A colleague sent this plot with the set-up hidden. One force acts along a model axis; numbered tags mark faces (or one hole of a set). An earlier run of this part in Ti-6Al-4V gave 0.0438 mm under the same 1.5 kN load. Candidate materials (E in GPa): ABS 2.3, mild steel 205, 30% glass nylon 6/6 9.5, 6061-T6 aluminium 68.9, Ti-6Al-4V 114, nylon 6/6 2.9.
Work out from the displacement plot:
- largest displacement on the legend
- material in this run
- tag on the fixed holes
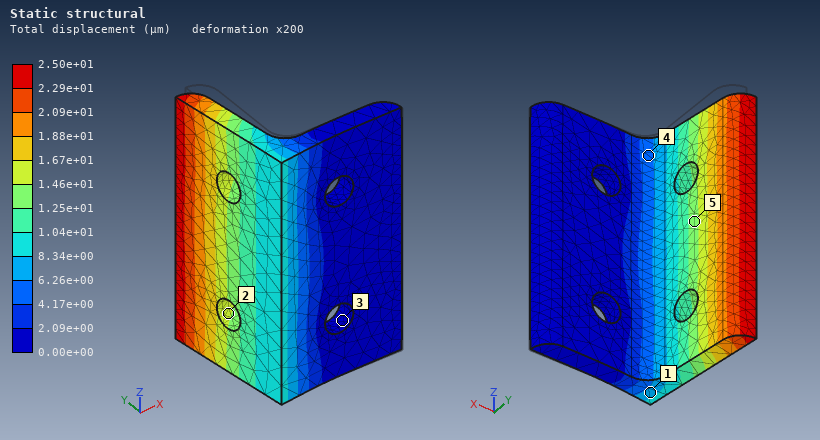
2.50e+01 µm
mild steel
3
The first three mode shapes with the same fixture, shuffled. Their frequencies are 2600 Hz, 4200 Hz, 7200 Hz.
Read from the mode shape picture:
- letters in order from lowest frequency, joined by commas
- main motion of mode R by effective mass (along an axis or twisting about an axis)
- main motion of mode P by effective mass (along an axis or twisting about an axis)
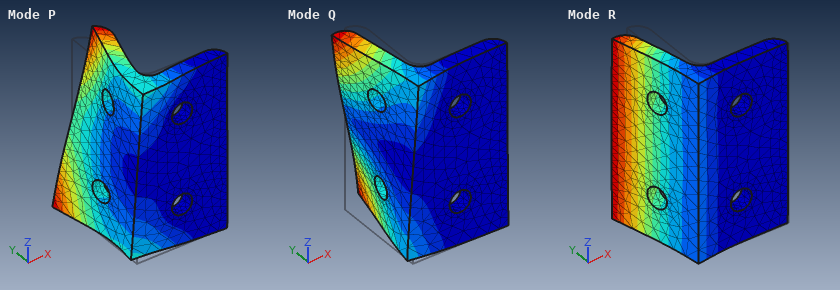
R, Q, P
along X
along Z
